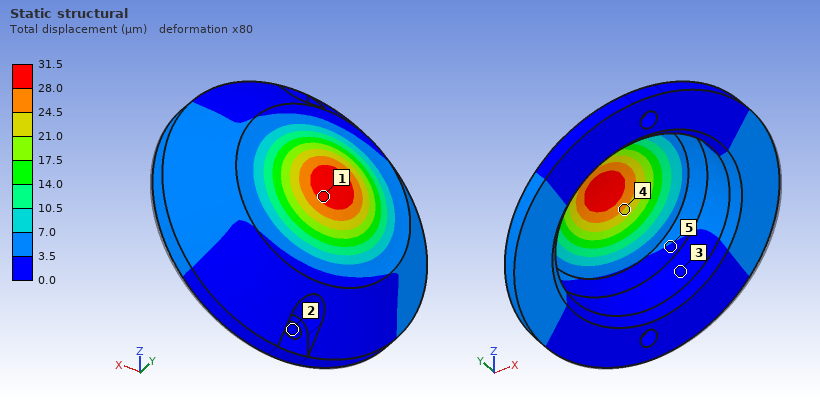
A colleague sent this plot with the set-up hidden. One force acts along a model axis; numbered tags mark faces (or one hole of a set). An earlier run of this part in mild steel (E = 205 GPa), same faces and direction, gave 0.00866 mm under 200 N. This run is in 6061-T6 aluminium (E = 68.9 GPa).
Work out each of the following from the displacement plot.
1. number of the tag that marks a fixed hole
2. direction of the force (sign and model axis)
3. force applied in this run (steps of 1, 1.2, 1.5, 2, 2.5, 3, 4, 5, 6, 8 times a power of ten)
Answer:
2
+Y
250 N
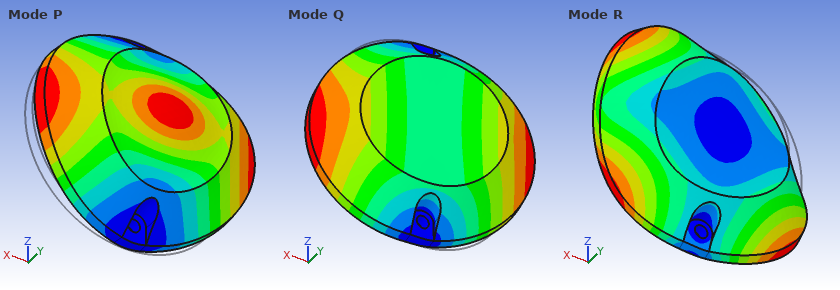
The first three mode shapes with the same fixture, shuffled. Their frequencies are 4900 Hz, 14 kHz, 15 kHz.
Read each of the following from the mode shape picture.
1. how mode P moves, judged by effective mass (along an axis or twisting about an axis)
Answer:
along Y
